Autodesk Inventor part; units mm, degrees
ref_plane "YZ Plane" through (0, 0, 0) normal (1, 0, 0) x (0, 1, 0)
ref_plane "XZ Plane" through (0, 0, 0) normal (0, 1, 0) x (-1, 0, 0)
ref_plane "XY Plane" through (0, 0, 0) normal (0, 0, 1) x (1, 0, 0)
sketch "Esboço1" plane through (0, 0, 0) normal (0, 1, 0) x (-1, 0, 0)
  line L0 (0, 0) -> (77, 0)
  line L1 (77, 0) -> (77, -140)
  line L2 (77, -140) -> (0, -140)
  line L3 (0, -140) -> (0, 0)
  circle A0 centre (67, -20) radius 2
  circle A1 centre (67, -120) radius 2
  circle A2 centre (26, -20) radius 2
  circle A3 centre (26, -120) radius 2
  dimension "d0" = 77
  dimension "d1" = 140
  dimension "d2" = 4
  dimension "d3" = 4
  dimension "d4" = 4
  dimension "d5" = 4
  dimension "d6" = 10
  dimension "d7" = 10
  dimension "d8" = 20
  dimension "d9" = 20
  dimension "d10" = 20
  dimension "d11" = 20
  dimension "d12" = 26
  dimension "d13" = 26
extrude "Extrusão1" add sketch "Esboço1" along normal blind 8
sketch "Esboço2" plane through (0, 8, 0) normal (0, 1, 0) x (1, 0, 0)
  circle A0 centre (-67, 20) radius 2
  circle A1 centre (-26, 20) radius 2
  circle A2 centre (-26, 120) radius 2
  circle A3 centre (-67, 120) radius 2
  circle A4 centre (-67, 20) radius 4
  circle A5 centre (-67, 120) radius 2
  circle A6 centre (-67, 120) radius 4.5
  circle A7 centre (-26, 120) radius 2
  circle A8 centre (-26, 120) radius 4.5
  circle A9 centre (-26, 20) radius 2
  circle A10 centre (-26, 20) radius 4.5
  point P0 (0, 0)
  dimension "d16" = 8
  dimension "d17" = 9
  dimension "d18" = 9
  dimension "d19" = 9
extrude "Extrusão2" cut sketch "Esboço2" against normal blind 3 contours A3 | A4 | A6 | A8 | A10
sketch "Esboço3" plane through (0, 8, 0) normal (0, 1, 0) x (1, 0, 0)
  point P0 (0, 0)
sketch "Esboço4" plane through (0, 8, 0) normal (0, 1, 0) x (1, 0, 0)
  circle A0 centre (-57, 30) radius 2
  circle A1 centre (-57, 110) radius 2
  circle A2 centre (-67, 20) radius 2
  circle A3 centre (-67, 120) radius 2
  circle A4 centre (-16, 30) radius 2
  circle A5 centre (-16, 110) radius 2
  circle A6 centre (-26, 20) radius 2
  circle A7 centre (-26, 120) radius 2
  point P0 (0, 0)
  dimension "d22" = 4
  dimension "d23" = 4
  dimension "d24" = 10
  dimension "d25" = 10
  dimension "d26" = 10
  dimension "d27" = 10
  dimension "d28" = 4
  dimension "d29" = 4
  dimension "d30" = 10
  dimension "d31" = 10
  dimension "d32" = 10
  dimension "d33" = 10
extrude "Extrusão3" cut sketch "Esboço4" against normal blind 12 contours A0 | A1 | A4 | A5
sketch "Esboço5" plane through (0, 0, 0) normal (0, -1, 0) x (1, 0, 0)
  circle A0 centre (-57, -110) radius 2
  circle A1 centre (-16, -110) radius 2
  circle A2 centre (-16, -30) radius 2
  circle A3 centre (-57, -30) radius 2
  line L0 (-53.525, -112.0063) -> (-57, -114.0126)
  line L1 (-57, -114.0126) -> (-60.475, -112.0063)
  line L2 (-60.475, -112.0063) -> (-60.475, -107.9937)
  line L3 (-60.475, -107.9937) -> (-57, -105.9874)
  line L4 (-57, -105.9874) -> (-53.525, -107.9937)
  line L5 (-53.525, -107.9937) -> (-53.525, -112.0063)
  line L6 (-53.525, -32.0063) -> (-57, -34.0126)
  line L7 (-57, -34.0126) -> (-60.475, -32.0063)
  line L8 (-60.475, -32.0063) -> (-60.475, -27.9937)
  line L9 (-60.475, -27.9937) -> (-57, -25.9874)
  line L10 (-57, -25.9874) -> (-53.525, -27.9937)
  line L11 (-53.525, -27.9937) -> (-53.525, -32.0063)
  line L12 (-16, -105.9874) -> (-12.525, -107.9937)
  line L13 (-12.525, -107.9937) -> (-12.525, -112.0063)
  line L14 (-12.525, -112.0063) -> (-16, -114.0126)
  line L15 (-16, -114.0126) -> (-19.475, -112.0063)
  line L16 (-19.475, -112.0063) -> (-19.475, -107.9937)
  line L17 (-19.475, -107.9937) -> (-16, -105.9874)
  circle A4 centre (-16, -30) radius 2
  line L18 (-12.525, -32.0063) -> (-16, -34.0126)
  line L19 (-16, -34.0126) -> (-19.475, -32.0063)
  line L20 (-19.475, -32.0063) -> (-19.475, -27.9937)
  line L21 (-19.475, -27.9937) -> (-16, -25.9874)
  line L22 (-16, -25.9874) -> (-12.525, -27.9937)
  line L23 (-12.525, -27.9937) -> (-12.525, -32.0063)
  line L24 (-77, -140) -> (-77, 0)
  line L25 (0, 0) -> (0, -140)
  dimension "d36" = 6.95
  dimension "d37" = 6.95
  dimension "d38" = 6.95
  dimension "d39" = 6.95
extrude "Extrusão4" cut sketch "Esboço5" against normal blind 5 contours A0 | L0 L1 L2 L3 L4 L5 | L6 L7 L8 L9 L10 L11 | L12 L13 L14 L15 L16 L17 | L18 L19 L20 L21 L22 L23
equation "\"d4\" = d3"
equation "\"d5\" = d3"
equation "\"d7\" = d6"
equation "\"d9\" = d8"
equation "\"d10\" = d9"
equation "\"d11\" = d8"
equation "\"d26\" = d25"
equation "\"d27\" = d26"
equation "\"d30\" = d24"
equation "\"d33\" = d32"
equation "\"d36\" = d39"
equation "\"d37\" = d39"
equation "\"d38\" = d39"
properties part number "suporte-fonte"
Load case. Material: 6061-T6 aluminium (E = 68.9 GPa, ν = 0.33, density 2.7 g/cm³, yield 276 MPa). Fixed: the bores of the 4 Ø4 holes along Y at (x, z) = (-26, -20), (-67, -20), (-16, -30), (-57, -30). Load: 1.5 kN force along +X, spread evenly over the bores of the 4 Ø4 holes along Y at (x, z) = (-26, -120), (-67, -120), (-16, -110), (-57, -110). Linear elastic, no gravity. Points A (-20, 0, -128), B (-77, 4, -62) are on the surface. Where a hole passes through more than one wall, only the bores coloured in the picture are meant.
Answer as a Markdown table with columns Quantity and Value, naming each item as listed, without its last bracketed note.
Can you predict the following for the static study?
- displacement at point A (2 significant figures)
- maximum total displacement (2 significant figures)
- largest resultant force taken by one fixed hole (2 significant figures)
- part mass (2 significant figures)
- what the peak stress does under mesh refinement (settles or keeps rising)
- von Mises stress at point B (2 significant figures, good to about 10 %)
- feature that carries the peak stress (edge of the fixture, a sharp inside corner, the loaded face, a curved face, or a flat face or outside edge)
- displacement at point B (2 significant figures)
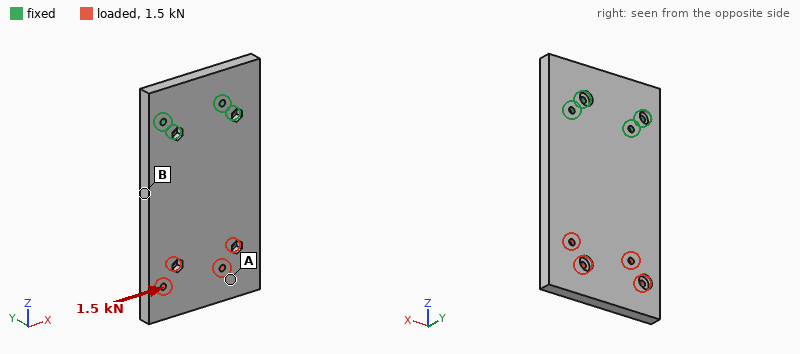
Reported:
| Quantity | Value |
|---|---|
| displacement at point A | 46 µm |
| maximum total displacement | 53 µm |
| largest resultant force taken by one fixed hole | 2.0 kN |
| part mass | 230 g |
| what the peak stress does under mesh refinement | keeps rising |
| von Mises stress at point B | 11 MPa |
| feature that carries the peak stress | edge of the fixture |
| displacement at point B | 17 µm |
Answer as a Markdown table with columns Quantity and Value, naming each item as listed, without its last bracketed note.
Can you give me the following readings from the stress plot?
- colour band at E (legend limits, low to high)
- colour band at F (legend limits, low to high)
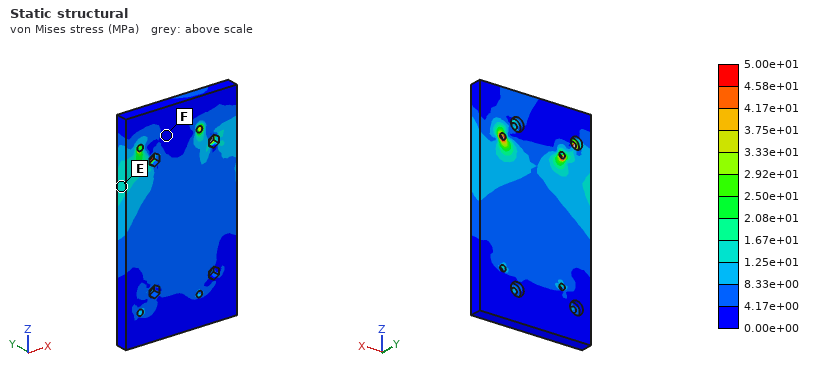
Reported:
| Quantity | Value |
|---|---|
| colour band at E | 1.25e+01 to 1.67e+01 MPa |
| colour band at F | 0.00e+00 to 4.17e+00 MPa |
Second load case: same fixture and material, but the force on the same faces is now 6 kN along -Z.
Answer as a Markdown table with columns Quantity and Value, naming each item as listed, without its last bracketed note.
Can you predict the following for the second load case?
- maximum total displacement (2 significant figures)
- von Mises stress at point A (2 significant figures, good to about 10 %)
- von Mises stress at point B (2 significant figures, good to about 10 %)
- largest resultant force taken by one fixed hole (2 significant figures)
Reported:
| Quantity | Value |
|---|---|
| maximum total displacement | 53 µm |
| von Mises stress at point A | 6.6 MPa |
| von Mises stress at point B | 12 MPa |
| largest resultant force taken by one fixed hole | 1.7 kN |
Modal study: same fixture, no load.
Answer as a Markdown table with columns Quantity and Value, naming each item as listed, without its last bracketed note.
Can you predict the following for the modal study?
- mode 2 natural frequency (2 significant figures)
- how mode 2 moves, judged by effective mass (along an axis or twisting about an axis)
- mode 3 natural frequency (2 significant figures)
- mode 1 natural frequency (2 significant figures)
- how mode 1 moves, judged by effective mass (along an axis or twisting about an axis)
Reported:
| Quantity | Value |
|---|---|
| mode 2 natural frequency | 1600 Hz |
| how mode 2 moves, judged by effective mass | twisting about Z |
| mode 3 natural frequency | 2900 Hz |
| mode 1 natural frequency | 490 Hz |
| how mode 1 moves, judged by effective mass | along Y |
